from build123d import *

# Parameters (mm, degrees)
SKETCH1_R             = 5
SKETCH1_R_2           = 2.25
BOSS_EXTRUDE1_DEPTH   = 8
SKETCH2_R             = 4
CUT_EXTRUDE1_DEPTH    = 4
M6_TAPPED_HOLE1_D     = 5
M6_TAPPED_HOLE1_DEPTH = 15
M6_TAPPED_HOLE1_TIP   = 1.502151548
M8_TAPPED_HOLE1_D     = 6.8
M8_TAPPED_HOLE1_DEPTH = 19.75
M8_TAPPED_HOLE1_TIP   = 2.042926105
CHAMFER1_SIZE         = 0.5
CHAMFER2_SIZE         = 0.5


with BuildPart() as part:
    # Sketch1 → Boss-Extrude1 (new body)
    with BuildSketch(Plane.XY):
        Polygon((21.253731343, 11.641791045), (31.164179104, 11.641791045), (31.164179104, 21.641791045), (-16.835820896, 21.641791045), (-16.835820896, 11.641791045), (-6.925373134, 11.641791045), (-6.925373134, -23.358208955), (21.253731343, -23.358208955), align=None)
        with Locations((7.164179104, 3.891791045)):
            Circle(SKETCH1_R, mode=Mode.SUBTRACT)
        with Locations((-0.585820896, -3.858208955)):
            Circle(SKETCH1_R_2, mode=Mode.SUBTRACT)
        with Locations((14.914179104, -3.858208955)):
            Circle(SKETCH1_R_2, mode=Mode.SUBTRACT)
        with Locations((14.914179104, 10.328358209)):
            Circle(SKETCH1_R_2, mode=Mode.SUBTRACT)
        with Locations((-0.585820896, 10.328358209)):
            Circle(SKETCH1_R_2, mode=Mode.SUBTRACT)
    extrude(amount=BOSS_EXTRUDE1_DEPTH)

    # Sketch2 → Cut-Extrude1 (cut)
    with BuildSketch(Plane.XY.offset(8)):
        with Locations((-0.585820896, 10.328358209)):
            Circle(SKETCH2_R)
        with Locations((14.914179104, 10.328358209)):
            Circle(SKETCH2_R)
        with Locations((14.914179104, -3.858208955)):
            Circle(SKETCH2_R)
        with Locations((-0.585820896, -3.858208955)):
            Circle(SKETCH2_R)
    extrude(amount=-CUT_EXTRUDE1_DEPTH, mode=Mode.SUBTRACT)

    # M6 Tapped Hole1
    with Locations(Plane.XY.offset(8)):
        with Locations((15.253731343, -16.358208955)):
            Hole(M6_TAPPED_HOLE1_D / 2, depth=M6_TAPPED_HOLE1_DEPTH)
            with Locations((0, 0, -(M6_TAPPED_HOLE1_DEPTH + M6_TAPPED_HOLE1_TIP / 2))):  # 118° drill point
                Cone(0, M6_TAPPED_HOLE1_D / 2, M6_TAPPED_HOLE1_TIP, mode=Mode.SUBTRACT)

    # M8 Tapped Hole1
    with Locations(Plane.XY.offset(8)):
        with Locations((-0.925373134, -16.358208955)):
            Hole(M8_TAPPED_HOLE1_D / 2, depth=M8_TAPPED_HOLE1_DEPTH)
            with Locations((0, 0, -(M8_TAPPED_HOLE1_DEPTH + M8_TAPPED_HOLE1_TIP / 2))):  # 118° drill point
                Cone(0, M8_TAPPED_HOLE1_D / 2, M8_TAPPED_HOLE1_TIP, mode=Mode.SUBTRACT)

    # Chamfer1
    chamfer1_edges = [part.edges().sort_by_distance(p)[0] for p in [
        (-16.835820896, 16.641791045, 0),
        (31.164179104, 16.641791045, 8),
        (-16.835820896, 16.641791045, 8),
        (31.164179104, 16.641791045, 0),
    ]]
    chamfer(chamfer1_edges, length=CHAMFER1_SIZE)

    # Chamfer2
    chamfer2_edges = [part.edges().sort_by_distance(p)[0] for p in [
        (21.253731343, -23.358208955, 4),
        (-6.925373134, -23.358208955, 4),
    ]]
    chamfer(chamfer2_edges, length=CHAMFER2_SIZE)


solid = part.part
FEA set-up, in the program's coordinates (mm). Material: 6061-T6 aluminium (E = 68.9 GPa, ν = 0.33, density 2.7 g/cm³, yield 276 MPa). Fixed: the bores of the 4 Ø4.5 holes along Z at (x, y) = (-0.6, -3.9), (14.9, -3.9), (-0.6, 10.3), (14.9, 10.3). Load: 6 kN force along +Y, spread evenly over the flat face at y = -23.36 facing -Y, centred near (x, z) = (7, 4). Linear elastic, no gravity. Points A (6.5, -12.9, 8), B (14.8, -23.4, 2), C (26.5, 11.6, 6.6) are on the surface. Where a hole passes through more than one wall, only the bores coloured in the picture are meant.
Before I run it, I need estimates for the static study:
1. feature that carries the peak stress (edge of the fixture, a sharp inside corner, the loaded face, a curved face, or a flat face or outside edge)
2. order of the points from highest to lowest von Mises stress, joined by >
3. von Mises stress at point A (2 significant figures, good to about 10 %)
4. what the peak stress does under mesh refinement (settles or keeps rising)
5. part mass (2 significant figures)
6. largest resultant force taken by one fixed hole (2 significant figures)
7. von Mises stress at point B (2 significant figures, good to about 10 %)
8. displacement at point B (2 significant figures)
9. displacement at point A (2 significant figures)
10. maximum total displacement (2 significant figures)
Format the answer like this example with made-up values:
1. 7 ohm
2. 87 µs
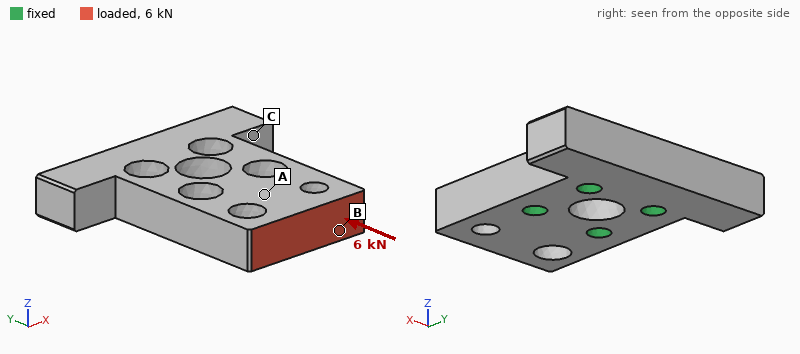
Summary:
1. edge of the fixture
2. A > B > C
3. 39 MPa
4. keeps rising
5. 26 g
6. 2.6 kN
7. 23 MPa
8. 26 µm
9. 18 µm
10. 34 µm
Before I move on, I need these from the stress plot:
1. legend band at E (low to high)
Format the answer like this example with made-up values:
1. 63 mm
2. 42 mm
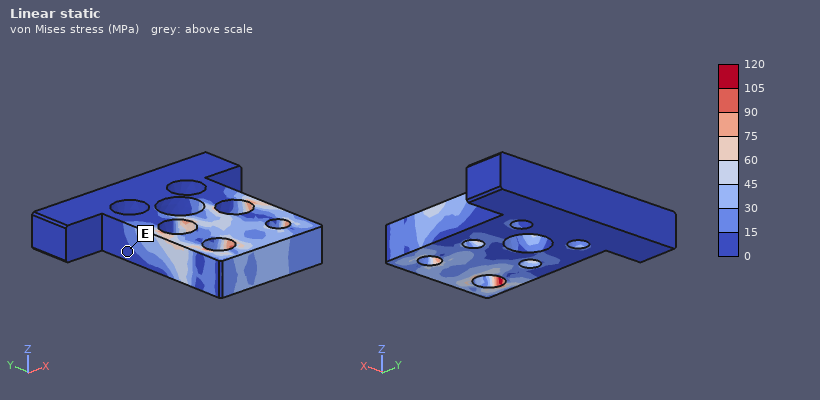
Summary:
1. 0 to 15 MPa
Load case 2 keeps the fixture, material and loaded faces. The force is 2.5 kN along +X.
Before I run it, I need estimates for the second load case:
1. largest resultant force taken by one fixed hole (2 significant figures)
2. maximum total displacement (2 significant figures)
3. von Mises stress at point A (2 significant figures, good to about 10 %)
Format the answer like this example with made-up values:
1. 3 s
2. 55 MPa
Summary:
1. 2.5 kN
2. 30 µm
3. 17 MPa
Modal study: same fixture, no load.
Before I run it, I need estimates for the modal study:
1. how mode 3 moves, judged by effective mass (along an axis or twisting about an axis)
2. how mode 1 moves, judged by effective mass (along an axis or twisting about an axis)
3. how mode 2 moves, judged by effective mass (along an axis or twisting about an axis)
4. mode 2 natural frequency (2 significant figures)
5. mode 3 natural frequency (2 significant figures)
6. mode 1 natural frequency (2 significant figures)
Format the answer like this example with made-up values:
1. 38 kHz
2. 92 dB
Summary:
1. along Z
2. along Z
3. twisting about Y
4. 15 kHz
5. 16 kHz
6. 11 kHz
